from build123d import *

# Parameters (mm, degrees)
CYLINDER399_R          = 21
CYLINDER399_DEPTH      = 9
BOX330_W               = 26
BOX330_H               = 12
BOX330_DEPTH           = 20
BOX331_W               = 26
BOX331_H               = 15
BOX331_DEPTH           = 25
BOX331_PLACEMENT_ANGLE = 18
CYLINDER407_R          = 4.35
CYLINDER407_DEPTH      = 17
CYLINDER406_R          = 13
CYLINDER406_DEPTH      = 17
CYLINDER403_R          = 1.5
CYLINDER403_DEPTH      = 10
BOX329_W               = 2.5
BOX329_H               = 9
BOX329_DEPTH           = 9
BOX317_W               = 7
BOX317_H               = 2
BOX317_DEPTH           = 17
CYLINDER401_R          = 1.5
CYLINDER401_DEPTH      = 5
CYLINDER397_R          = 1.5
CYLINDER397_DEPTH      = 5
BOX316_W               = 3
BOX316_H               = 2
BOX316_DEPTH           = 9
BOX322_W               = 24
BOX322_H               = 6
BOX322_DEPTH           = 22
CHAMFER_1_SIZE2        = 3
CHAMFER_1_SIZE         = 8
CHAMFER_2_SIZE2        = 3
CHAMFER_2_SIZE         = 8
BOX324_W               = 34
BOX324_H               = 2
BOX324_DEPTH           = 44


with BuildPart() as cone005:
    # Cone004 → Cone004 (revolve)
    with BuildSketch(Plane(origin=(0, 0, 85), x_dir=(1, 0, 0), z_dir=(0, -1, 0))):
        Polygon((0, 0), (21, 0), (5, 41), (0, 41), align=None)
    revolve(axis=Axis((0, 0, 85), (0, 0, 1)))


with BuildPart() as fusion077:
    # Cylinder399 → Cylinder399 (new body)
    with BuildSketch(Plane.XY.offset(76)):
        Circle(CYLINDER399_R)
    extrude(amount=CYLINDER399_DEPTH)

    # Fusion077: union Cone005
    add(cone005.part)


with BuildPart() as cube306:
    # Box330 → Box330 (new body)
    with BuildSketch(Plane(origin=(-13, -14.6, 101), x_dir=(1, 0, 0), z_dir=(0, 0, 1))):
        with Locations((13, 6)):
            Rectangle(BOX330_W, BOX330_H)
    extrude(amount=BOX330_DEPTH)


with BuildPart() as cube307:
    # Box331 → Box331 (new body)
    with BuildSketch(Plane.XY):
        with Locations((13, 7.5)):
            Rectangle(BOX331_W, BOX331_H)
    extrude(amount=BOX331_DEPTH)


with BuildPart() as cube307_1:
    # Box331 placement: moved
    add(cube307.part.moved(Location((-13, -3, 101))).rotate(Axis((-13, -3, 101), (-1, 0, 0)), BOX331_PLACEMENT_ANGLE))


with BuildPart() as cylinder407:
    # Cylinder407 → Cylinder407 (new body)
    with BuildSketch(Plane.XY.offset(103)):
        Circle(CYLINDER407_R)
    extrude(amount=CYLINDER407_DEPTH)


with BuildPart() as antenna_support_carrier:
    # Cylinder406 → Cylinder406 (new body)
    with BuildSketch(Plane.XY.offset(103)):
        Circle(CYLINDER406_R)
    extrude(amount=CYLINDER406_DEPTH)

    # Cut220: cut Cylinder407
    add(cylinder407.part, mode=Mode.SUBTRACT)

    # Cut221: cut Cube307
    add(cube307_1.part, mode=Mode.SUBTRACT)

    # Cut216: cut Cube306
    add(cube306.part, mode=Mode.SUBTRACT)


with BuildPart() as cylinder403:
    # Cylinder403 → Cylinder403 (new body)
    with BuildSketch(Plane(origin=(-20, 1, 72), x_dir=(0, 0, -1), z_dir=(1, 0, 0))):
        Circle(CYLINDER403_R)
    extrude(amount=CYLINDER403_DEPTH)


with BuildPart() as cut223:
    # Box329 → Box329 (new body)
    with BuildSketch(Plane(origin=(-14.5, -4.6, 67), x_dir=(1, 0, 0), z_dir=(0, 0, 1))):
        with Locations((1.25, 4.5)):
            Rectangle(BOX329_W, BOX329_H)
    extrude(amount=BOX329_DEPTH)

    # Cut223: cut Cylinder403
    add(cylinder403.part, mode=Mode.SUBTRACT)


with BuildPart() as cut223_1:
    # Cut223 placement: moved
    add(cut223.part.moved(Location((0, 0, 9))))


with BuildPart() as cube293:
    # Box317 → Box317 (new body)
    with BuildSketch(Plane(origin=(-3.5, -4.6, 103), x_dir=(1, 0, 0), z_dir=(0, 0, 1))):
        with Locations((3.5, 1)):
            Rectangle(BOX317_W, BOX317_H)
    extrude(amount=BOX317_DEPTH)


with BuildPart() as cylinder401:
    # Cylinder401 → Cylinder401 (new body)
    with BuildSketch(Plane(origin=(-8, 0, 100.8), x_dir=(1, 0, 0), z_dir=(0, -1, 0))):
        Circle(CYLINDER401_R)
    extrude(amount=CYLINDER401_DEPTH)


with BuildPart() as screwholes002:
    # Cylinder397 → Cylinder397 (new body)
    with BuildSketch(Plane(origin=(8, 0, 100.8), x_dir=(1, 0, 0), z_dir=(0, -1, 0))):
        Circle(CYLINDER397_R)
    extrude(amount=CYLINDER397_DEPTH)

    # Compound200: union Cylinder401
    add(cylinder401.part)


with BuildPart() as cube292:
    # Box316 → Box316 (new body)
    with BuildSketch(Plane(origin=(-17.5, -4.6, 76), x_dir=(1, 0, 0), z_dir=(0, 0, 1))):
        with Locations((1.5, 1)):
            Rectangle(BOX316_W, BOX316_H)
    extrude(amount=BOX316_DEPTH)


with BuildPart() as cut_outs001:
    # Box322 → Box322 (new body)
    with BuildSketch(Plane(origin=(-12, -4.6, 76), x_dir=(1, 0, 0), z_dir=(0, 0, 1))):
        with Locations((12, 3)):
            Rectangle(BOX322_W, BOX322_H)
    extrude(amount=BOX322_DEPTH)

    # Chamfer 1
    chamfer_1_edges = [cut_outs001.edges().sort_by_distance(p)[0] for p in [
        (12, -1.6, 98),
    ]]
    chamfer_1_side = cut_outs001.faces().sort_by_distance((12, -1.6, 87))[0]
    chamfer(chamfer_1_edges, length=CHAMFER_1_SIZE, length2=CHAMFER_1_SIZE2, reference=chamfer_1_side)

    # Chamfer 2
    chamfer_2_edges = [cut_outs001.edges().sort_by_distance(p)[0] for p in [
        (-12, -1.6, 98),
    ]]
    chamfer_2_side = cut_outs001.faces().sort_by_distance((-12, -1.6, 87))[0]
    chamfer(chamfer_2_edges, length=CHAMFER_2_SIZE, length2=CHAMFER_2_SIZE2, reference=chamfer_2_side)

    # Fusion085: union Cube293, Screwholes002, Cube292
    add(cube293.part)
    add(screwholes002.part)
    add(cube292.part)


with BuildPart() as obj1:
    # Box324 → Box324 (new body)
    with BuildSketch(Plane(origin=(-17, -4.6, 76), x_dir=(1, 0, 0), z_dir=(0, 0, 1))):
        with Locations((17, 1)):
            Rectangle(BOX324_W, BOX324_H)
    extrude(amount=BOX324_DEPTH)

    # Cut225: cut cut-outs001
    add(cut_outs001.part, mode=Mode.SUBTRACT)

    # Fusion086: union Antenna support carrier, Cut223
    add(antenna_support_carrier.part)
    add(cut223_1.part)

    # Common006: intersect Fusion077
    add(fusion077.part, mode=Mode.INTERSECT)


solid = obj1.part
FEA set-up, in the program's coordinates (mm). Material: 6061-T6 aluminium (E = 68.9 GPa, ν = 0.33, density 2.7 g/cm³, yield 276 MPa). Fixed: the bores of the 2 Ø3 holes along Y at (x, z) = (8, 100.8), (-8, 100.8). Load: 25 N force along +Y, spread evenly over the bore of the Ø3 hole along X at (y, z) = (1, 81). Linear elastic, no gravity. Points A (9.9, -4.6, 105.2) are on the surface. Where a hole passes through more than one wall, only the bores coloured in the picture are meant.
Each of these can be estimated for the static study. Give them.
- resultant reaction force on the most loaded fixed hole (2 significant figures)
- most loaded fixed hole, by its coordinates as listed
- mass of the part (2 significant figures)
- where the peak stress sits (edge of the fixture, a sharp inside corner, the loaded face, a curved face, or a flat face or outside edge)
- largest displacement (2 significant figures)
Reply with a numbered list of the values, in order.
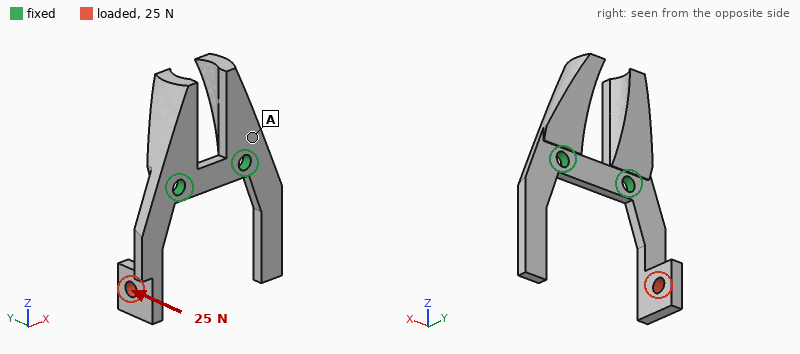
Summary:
1. 24 N
2. (-8, 100.8)
3. 4.9 g
4. a flat face or outside edge
5. 0.40 mm
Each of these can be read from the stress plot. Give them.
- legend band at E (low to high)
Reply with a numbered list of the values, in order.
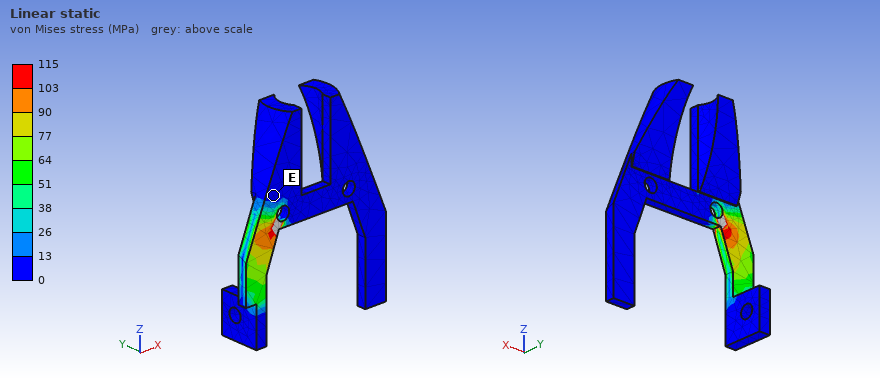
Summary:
1. 0 to 13 MPa
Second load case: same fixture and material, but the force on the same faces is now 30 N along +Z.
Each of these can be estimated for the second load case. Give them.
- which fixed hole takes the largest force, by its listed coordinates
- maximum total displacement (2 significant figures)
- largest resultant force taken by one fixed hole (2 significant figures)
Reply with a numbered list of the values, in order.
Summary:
1. (-8, 100.8)
2. 0.19 mm
3. 32 N
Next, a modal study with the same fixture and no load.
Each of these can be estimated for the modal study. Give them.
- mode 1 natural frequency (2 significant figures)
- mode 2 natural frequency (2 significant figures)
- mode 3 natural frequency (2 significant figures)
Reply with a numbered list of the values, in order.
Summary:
1. 1900 Hz
2. 2700 Hz
3. 4000 Hz
